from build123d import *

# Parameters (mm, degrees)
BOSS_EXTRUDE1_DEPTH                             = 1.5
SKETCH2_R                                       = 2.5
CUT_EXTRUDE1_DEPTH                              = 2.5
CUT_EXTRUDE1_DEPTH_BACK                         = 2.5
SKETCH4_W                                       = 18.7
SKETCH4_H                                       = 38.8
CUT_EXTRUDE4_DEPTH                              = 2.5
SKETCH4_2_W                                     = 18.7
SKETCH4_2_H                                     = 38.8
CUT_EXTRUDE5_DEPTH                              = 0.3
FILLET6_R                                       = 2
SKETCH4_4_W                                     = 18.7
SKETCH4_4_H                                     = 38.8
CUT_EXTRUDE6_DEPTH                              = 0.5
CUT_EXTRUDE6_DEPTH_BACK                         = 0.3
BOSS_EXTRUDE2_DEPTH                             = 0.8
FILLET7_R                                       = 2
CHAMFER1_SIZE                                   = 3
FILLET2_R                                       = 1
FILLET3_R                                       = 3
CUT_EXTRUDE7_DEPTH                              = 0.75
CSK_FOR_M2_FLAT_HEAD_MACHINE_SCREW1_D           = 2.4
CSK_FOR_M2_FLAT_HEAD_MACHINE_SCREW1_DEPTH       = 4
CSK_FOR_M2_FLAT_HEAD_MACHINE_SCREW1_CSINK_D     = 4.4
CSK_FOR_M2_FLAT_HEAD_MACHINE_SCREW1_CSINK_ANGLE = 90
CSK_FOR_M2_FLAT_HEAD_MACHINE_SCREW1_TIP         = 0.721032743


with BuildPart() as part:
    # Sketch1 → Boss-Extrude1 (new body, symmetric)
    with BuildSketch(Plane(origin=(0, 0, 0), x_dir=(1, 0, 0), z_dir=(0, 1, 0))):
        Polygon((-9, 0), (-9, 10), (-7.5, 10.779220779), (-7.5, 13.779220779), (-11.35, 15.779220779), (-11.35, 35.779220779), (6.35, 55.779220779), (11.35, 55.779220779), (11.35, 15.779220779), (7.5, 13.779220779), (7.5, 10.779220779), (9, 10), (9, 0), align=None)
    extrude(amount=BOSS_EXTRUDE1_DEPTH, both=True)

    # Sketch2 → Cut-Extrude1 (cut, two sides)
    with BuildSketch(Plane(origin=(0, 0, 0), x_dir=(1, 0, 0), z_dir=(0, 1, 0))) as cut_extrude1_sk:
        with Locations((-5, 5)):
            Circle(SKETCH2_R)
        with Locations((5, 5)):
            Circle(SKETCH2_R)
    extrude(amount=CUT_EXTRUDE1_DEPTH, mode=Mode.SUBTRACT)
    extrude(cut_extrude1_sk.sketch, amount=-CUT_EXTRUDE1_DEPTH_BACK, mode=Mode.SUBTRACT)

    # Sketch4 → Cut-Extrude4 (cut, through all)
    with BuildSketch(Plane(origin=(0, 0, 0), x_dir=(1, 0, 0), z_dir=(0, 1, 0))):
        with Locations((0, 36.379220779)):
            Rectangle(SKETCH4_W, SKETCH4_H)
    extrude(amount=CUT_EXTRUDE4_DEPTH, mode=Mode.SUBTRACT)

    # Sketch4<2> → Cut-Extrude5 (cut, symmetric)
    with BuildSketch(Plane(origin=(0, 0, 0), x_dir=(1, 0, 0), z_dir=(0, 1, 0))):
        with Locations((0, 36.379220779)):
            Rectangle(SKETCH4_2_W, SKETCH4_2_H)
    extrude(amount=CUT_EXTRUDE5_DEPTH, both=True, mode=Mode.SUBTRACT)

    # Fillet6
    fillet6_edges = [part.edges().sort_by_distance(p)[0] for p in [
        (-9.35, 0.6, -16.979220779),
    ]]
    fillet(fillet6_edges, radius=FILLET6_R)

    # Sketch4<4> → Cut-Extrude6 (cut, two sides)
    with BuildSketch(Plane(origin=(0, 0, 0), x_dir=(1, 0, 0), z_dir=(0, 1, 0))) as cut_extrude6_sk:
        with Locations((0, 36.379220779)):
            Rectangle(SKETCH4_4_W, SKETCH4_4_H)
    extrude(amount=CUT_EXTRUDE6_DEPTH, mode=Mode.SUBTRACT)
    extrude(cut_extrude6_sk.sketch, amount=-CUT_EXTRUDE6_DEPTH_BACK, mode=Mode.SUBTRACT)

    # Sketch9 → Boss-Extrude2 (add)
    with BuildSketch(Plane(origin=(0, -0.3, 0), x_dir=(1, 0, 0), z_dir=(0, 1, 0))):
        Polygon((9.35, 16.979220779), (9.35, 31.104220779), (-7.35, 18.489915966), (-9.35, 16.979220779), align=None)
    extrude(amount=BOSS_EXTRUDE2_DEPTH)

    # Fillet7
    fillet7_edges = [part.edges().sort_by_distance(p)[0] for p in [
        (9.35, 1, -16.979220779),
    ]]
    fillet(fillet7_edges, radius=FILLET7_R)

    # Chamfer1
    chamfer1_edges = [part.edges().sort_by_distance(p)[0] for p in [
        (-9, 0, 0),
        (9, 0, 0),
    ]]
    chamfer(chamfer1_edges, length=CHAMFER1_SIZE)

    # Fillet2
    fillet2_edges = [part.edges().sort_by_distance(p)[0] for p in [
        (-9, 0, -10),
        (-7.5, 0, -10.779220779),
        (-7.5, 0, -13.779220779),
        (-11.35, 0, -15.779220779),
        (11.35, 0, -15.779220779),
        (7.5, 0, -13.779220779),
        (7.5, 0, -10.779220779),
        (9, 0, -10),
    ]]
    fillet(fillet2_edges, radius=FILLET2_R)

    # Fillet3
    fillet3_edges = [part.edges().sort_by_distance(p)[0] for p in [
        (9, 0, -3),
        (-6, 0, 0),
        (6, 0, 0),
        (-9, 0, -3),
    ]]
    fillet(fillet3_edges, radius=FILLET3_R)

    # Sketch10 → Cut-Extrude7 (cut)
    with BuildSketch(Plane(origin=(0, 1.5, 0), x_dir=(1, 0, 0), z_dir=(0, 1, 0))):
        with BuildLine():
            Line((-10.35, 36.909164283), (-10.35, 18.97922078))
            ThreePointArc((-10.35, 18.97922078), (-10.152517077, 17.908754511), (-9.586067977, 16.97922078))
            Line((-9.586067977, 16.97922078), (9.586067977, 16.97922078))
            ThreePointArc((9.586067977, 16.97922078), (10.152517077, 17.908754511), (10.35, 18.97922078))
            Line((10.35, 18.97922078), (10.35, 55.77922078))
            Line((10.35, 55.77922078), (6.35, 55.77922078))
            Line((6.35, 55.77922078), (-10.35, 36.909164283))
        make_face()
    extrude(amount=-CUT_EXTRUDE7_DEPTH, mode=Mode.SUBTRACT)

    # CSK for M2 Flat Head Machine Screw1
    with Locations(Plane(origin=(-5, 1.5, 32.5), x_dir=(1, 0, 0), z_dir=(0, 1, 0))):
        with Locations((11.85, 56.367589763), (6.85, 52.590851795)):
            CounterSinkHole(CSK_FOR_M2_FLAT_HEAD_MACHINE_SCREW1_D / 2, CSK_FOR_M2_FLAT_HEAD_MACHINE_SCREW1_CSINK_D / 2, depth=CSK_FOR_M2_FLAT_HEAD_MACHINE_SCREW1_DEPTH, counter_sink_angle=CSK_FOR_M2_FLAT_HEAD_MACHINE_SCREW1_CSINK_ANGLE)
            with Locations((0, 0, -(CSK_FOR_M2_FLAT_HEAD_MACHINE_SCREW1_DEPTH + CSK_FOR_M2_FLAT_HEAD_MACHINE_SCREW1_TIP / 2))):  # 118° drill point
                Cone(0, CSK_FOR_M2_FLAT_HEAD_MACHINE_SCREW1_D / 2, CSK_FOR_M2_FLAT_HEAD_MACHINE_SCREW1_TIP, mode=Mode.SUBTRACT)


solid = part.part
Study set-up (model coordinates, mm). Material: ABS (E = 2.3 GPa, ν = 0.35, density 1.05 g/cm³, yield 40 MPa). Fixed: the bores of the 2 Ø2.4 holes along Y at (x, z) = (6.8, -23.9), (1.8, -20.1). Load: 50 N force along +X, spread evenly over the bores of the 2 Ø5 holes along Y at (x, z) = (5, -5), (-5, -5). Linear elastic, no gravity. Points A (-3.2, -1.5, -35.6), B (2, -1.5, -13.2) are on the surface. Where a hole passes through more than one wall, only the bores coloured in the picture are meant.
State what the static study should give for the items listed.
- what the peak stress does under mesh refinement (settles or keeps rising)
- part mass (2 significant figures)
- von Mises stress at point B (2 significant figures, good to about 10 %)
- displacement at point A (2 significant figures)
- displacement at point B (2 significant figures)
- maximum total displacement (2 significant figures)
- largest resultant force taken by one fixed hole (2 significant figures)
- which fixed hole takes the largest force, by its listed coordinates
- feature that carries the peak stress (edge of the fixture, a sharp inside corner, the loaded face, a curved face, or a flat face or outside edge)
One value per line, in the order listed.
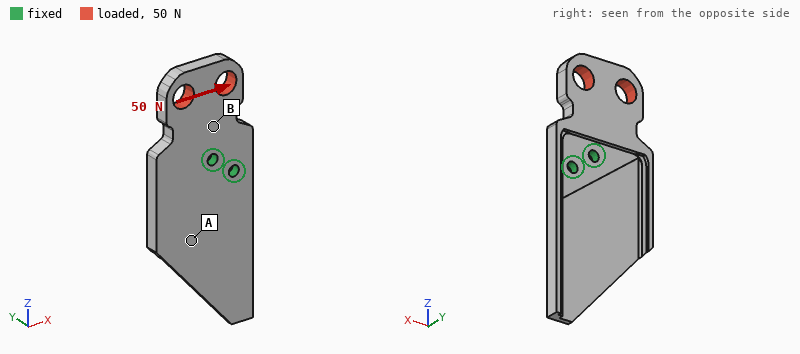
keeps rising
2.0 g
3.2 MPa
0.072 mm
0.048 mm
0.18 mm
120 N
(1.8, -20.1)
edge of the fixture
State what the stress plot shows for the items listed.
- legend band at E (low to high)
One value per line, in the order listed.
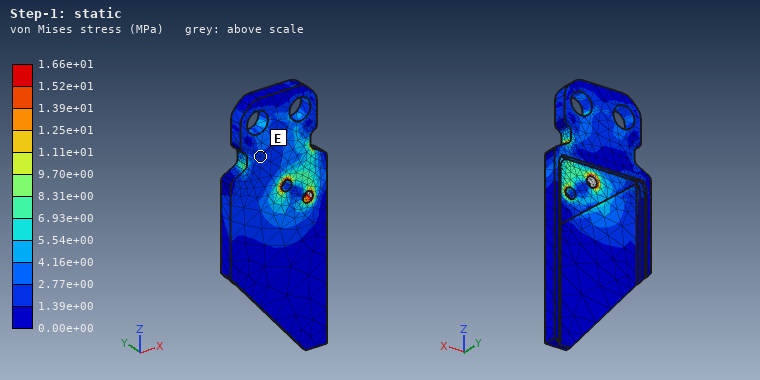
1.39e+00 to 2.77e+00 MPa
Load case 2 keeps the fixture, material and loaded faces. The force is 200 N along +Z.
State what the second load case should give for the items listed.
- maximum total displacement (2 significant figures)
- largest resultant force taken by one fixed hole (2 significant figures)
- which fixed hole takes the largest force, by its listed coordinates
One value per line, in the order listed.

0.32 mm
210 N
(1.8, -20.1)
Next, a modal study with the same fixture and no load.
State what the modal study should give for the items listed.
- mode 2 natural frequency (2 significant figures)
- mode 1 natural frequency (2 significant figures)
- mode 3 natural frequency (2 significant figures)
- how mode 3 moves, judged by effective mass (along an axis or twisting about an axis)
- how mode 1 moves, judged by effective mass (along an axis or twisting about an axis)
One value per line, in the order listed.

1200 Hz
620 Hz
1500 Hz
along Y
along Y
